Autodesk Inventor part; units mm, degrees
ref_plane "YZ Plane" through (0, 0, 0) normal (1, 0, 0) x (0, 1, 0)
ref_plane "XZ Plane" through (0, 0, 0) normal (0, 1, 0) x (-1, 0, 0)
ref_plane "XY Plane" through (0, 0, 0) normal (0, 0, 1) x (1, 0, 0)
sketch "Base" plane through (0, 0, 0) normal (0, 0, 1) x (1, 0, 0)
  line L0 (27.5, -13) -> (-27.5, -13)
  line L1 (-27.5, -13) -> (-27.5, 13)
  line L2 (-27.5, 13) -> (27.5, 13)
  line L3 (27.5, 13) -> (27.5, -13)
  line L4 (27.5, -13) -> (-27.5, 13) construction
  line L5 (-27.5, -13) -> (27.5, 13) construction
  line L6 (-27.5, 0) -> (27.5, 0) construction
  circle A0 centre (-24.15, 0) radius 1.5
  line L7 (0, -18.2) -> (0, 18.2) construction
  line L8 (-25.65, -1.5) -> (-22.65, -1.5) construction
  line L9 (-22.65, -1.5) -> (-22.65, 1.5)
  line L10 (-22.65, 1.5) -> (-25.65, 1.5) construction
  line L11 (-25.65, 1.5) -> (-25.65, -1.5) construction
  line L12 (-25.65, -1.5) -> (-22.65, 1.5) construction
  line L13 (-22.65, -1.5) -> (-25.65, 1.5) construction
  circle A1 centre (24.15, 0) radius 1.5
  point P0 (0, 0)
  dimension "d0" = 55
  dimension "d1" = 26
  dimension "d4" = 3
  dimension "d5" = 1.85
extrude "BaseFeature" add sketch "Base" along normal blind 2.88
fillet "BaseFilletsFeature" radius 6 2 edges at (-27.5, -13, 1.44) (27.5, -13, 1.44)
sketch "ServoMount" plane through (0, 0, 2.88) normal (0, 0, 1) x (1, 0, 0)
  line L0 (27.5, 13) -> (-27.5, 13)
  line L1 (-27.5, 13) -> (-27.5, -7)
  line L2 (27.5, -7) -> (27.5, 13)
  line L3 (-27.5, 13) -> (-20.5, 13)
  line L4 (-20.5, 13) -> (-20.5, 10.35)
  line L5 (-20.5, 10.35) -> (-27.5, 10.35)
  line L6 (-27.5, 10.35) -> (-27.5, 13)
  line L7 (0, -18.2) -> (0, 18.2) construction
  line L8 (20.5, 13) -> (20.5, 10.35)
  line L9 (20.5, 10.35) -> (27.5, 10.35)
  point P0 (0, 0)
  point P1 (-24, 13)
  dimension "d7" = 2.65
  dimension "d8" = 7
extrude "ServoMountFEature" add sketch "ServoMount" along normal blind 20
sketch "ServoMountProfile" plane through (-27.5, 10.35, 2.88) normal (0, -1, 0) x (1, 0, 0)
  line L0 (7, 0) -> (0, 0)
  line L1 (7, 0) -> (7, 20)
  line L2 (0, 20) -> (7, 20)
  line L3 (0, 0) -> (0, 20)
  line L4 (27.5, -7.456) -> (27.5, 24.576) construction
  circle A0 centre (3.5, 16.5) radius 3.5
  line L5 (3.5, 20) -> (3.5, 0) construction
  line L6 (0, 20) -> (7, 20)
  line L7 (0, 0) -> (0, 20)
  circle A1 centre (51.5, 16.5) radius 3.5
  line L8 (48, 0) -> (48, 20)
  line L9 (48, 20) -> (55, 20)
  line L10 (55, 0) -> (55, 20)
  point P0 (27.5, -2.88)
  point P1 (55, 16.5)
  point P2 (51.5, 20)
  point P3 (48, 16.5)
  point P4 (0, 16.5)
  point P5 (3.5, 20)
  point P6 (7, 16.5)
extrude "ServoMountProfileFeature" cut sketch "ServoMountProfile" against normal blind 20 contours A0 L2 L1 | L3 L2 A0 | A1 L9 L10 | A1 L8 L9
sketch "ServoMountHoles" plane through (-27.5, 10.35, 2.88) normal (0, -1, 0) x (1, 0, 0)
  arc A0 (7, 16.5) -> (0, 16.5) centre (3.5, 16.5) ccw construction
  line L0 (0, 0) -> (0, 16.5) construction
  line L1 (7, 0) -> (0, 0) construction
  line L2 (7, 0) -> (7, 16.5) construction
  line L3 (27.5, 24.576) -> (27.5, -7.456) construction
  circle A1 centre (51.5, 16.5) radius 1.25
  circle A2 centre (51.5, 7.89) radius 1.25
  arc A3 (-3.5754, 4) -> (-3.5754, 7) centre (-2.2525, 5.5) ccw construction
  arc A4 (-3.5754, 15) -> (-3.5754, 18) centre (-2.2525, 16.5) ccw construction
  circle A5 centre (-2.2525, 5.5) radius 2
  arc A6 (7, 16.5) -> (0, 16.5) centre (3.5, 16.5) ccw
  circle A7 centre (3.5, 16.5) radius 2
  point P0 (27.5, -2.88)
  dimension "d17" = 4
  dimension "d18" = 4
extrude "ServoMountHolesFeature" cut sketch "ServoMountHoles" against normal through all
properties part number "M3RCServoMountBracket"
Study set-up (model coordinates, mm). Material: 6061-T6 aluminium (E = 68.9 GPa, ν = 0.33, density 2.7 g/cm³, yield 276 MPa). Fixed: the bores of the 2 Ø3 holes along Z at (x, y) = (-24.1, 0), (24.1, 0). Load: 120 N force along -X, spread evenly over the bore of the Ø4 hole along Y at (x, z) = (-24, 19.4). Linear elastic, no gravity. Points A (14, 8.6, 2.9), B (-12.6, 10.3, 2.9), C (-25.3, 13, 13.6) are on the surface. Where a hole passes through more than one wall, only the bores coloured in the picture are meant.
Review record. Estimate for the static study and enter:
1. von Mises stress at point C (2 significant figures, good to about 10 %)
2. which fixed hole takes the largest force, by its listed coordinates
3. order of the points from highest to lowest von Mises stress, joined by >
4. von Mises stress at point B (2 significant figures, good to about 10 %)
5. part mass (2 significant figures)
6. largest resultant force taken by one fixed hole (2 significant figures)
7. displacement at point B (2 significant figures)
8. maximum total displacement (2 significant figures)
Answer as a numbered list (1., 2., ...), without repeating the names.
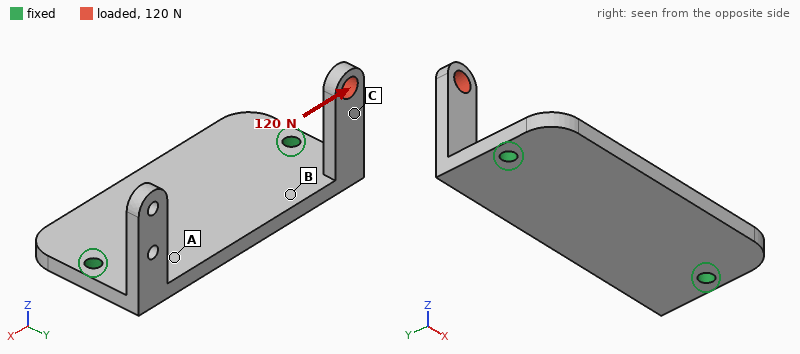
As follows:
1. 18 MPa
2. (-24.1, 0)
3. B > C > A
4. 36 MPa
5. 13 g
6. 87 N
7. 0.038 mm
8. 0.25 mm
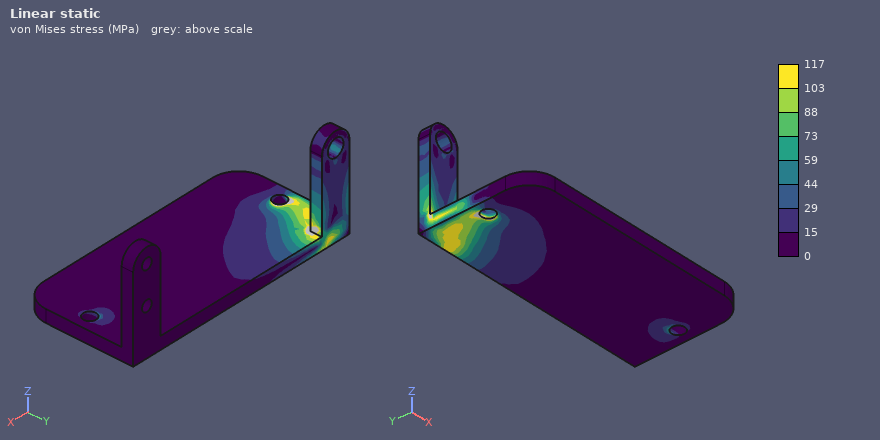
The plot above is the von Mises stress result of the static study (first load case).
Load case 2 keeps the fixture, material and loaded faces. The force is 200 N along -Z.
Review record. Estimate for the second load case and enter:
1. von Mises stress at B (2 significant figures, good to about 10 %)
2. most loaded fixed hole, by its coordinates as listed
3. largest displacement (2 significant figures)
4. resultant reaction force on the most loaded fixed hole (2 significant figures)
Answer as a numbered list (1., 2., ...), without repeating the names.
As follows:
1. 26 MPa
2. (-24.1, 0)
3. 0.16 mm
4. 200 N
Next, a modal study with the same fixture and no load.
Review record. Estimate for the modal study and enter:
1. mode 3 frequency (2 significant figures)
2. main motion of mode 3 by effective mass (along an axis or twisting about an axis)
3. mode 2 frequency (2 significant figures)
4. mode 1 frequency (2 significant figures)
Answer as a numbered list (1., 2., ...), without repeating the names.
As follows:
1. 4700 Hz
2. along Z
3. 4000 Hz
4. 3700 Hz
